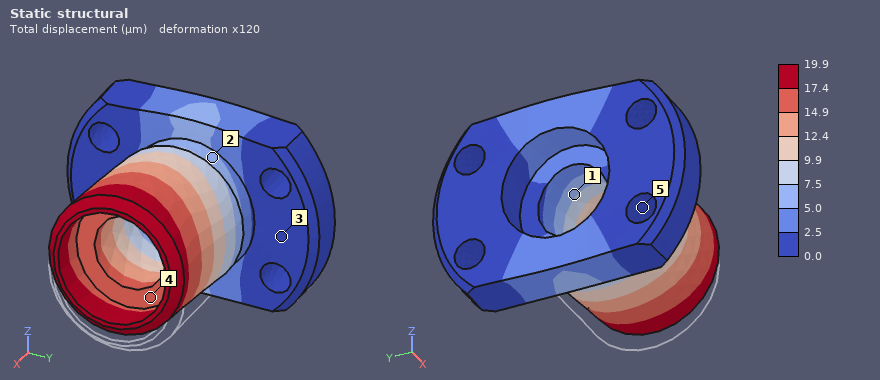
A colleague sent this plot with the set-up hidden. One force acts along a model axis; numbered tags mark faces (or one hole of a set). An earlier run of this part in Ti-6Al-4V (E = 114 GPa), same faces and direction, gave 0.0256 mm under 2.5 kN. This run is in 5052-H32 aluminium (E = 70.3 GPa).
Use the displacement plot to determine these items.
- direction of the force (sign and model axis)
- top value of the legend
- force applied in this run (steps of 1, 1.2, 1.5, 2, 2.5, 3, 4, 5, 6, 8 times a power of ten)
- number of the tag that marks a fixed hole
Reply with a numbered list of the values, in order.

1. +Z
2. 19.9 µm
3. 1.2 kN
4. 5
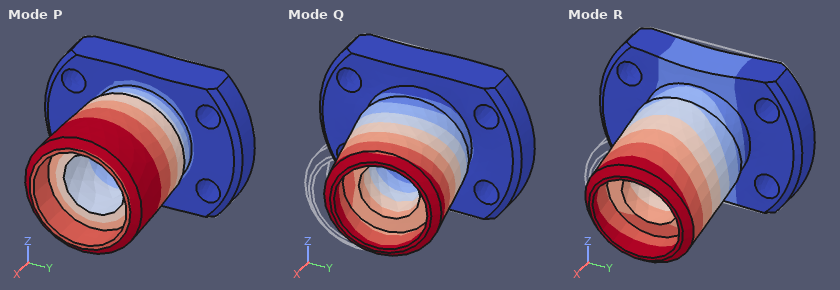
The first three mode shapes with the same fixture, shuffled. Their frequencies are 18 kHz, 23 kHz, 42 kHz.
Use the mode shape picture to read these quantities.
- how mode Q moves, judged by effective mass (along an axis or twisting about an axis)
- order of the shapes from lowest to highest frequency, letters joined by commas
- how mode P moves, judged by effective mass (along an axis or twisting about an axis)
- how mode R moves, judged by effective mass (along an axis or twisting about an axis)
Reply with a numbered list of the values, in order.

1. along Y
2. R, Q, P
3. twisting about X
4. along Z
